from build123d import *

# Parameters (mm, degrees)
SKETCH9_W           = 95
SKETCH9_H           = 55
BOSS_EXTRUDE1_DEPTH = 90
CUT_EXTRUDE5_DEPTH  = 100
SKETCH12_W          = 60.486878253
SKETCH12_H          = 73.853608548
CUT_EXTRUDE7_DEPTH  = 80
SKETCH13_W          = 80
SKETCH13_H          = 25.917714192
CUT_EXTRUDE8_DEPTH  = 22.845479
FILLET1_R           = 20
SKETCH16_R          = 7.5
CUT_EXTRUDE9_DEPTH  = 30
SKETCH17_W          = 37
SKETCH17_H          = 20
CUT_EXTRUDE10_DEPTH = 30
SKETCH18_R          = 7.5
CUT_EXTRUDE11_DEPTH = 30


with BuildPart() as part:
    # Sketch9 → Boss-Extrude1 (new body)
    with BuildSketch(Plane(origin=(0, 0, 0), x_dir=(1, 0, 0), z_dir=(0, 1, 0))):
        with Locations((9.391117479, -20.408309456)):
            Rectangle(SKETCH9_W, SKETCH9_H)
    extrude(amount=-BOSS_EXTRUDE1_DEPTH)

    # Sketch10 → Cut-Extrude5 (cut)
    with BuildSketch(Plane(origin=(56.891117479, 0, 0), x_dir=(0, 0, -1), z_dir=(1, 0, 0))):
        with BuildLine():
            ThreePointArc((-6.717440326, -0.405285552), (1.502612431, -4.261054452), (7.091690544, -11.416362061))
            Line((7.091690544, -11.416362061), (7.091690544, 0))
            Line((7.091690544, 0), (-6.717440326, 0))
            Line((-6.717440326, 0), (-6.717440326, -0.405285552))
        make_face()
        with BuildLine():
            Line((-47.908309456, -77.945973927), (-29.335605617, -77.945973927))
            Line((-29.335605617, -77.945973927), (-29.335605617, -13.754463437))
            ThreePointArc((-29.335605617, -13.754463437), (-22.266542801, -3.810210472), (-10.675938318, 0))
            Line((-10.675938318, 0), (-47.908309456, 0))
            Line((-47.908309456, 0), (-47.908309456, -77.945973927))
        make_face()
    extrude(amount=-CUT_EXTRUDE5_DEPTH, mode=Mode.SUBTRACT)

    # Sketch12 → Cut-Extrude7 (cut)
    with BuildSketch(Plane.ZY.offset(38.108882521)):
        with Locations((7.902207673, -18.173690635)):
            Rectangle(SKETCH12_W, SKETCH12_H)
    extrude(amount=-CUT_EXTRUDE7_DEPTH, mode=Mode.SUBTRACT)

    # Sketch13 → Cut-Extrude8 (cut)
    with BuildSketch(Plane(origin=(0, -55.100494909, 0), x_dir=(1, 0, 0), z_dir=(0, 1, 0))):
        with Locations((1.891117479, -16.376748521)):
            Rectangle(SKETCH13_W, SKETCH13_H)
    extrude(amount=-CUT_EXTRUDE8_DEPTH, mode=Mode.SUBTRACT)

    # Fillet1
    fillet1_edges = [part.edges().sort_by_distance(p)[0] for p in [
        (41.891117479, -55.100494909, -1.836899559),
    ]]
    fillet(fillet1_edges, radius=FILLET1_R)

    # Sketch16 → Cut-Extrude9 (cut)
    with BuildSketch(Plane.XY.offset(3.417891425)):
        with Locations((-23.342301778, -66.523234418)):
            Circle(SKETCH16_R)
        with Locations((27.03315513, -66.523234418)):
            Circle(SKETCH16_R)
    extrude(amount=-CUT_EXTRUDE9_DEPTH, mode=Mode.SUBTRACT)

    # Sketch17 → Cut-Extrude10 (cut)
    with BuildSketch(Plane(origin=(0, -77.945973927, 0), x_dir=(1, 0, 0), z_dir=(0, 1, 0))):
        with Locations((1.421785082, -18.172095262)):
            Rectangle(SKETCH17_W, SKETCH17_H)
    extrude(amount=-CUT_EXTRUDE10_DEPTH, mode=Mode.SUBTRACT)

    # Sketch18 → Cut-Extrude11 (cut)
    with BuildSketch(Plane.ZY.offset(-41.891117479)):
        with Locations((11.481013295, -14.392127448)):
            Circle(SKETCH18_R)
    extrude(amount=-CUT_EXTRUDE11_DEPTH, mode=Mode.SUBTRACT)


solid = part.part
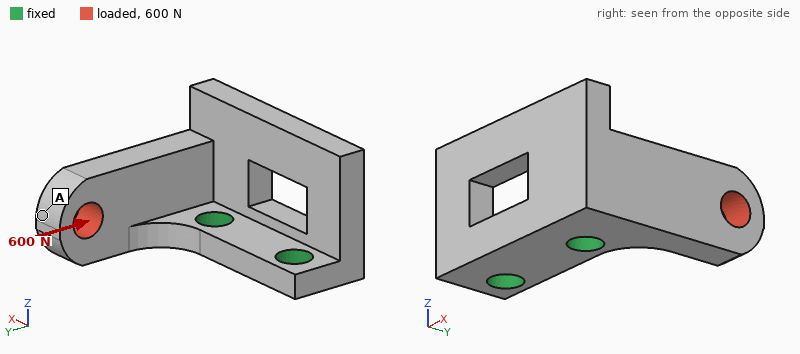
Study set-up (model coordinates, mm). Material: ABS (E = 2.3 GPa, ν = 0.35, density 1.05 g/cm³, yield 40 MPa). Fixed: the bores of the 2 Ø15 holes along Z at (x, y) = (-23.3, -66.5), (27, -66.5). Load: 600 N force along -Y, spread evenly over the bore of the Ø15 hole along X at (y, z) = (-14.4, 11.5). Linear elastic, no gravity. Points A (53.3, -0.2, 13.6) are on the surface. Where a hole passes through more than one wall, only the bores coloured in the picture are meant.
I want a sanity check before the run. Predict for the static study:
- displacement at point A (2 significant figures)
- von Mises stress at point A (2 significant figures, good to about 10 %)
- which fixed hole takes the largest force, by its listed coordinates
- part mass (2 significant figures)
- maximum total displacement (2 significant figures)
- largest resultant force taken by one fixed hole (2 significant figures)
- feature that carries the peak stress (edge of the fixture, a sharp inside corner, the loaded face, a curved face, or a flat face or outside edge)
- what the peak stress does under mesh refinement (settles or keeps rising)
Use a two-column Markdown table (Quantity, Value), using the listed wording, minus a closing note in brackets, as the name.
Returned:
| Quantity | Value |
|---|---|
| displacement at point A | 0.38 mm |
| von Mises stress at point A | 1.9 MPa |
| which fixed hole takes the largest force, by its listed coordinates | (27, -66.5) |
| part mass | 110 g |
| maximum total displacement | 0.39 mm |
| largest resultant force taken by one fixed hole | 690 N |
| feature that carries the peak stress | edge of the fixture |
| what the peak stress does under mesh refinement | keeps rising |
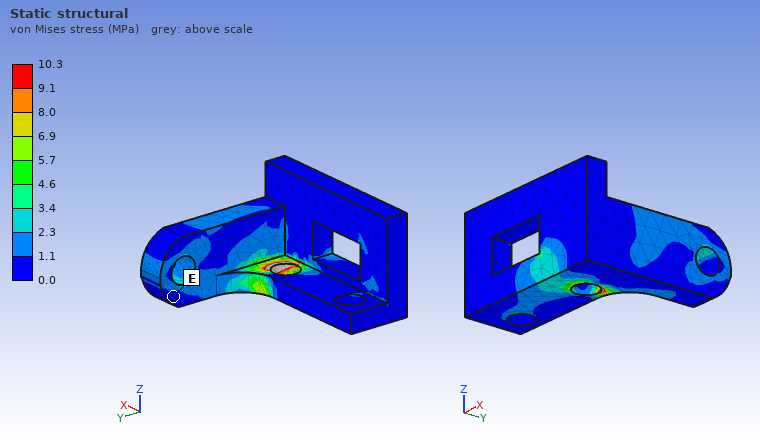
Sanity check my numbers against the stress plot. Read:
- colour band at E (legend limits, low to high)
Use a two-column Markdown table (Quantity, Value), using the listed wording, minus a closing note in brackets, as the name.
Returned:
| Quantity | Value |
|---|---|
| colour band at E | 0.0 to 1.1 MPa |
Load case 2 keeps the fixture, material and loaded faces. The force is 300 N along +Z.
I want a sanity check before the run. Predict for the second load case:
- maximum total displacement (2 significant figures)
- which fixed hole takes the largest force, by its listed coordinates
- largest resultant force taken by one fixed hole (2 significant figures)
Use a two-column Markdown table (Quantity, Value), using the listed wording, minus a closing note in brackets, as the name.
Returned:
| Quantity | Value |
|---|---|
| maximum total displacement | 0.88 mm |
| which fixed hole takes the largest force, by its listed coordinates | (27, -66.5) |
| largest resultant force taken by one fixed hole | 300 N |
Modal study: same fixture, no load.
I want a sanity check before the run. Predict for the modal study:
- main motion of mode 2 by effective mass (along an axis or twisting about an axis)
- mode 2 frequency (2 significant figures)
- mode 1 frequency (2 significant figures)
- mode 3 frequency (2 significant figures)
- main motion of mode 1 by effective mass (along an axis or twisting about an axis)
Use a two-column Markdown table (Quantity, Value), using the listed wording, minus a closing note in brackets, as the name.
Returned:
| Quantity | Value |
|---|---|
| main motion of mode 2 by effective mass | along X |
| mode 2 frequency | 850 Hz |
| mode 1 frequency | 650 Hz |
| mode 3 frequency | 1000 Hz |
| main motion of mode 1 by effective mass | along Y |
